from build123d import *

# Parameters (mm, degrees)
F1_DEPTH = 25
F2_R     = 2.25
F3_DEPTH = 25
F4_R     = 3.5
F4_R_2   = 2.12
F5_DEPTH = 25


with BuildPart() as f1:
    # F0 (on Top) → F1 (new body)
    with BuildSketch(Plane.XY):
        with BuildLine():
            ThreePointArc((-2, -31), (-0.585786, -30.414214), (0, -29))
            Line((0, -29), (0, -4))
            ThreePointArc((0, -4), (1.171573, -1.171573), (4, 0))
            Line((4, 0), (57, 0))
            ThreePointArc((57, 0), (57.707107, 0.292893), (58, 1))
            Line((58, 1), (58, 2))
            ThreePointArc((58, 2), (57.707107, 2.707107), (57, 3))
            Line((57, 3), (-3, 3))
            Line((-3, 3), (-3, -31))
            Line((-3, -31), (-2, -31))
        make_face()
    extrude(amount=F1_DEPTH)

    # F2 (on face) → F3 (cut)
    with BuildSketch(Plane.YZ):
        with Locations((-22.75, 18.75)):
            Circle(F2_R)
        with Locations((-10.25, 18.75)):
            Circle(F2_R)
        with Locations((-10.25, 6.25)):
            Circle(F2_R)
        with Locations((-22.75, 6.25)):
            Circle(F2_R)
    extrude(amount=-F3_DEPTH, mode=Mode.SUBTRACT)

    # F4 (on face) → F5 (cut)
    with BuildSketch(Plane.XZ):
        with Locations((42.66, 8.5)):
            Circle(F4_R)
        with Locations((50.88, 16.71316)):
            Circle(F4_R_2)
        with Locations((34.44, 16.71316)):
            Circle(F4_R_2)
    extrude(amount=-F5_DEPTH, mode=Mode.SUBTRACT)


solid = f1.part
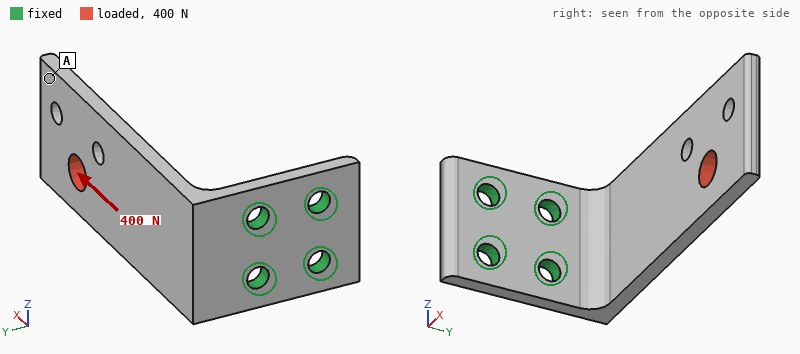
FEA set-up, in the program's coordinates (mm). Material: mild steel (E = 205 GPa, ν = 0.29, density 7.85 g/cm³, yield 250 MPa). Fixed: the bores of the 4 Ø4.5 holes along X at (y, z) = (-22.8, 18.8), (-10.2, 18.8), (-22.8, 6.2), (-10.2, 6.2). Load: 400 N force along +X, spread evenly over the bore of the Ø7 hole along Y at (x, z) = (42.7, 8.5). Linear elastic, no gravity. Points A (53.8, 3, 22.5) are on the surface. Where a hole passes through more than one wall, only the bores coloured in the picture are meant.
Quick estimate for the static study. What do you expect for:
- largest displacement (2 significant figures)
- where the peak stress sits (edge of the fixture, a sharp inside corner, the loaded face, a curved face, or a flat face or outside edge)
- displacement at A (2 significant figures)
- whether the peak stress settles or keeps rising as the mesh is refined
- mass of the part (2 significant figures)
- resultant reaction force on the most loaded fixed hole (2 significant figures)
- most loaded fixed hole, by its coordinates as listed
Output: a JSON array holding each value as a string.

["0.11 mm", "edge of the fixture", "0.097 mm", "keeps rising", "52 g", "310 N", "(-10.2, 6.2)"]
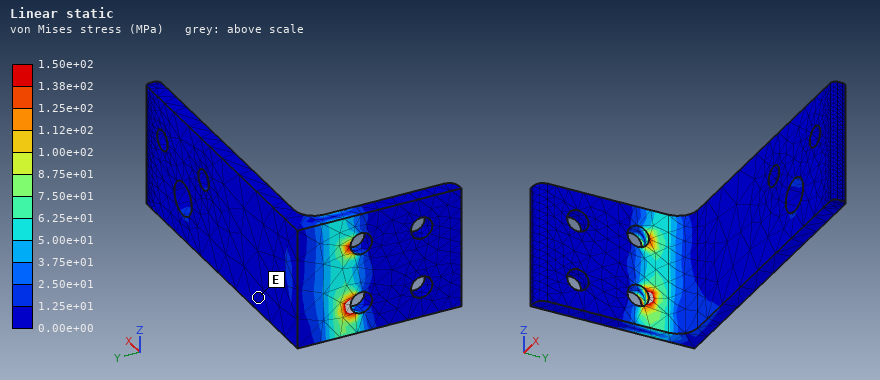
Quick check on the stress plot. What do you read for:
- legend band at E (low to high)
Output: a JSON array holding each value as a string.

["0.00e+00 to 1.25e+01 MPa"]
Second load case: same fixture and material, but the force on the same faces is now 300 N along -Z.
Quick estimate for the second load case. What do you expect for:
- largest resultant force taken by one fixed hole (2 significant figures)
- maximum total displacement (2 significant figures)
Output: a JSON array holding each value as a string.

["860 N", "0.16 mm"]
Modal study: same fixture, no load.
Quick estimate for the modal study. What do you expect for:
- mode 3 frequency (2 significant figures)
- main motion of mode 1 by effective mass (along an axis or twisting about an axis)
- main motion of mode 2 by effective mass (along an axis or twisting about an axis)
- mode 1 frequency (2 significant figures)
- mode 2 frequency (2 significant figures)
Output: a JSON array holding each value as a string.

["3500 Hz", "along Y", "along Z", "630 Hz", "1800 Hz"]
